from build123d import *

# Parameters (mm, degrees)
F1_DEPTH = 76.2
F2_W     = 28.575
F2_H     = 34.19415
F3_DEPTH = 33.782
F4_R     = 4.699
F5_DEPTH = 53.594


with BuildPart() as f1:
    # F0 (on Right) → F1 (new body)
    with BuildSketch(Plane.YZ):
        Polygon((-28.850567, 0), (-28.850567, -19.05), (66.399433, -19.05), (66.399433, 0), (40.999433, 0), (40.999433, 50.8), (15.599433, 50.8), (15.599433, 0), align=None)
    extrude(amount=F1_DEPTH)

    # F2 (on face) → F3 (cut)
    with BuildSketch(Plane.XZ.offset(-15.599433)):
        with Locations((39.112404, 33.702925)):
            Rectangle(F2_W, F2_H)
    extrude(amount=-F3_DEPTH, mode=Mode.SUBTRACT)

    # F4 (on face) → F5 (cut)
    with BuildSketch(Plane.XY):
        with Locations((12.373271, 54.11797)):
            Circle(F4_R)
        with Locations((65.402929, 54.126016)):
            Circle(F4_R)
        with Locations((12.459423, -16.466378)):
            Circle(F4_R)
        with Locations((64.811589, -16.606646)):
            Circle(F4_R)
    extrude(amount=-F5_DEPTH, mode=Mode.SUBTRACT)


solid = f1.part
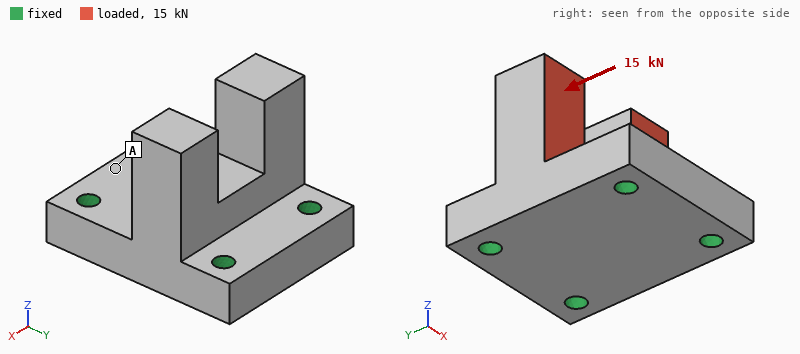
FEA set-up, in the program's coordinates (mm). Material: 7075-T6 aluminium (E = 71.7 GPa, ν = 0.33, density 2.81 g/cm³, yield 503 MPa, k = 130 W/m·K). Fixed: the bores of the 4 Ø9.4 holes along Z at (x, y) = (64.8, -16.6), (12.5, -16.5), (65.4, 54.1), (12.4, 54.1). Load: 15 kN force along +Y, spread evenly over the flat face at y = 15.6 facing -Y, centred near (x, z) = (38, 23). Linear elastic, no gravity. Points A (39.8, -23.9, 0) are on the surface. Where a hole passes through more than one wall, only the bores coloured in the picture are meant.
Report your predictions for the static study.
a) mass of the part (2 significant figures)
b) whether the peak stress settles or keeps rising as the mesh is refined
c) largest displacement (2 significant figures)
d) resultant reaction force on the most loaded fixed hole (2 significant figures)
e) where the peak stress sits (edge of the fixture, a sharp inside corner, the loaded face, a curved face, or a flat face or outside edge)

580 g
keeps rising
96 µm
6.2 kN
edge of the fixture
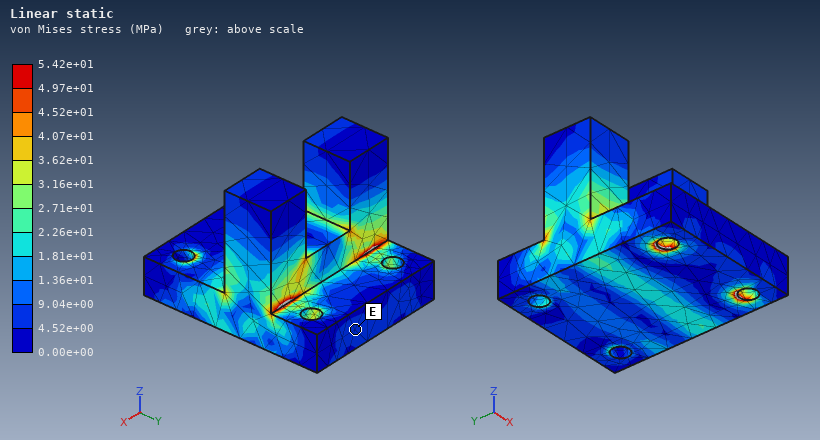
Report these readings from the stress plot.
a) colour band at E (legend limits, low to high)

4.52e+00 to 9.04e+00 MPa
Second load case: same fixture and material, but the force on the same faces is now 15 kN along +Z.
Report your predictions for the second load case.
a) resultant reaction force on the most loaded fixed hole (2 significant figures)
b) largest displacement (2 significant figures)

4.4 kN
67 µm
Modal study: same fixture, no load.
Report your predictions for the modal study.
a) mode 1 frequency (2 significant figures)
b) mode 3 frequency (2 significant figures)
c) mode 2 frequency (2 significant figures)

5400 Hz
6300 Hz
5600 Hz
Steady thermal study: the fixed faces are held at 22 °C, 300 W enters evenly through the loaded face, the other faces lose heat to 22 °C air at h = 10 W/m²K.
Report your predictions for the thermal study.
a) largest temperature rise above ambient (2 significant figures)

69 K
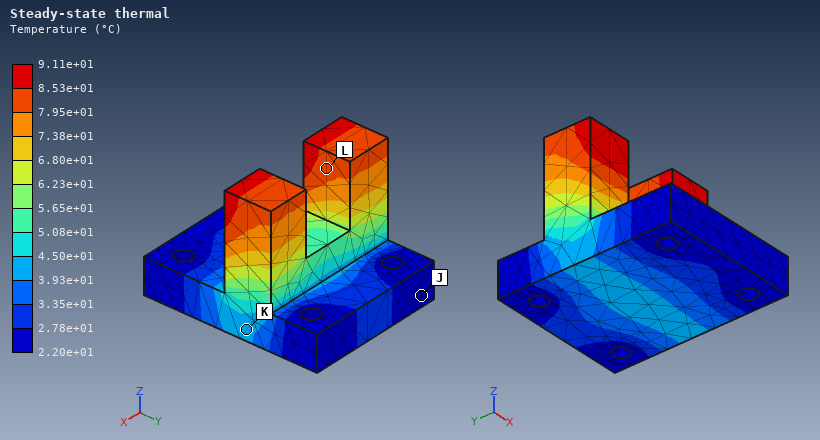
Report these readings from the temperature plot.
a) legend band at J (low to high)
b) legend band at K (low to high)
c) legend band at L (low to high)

2.20e+01 to 2.78e+01 °C
3.93e+01 to 4.50e+01 °C
7.95e+01 to 8.53e+01 °C
